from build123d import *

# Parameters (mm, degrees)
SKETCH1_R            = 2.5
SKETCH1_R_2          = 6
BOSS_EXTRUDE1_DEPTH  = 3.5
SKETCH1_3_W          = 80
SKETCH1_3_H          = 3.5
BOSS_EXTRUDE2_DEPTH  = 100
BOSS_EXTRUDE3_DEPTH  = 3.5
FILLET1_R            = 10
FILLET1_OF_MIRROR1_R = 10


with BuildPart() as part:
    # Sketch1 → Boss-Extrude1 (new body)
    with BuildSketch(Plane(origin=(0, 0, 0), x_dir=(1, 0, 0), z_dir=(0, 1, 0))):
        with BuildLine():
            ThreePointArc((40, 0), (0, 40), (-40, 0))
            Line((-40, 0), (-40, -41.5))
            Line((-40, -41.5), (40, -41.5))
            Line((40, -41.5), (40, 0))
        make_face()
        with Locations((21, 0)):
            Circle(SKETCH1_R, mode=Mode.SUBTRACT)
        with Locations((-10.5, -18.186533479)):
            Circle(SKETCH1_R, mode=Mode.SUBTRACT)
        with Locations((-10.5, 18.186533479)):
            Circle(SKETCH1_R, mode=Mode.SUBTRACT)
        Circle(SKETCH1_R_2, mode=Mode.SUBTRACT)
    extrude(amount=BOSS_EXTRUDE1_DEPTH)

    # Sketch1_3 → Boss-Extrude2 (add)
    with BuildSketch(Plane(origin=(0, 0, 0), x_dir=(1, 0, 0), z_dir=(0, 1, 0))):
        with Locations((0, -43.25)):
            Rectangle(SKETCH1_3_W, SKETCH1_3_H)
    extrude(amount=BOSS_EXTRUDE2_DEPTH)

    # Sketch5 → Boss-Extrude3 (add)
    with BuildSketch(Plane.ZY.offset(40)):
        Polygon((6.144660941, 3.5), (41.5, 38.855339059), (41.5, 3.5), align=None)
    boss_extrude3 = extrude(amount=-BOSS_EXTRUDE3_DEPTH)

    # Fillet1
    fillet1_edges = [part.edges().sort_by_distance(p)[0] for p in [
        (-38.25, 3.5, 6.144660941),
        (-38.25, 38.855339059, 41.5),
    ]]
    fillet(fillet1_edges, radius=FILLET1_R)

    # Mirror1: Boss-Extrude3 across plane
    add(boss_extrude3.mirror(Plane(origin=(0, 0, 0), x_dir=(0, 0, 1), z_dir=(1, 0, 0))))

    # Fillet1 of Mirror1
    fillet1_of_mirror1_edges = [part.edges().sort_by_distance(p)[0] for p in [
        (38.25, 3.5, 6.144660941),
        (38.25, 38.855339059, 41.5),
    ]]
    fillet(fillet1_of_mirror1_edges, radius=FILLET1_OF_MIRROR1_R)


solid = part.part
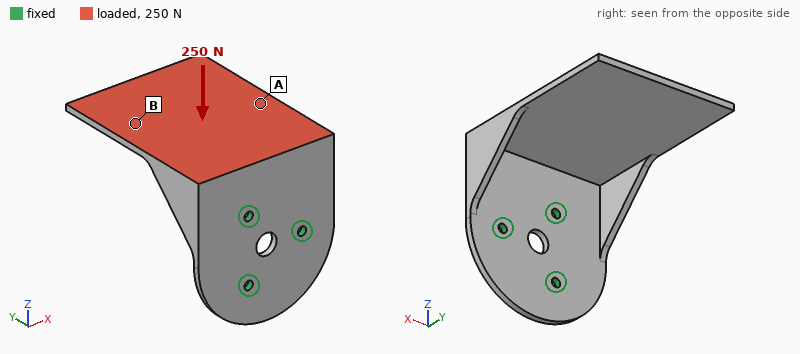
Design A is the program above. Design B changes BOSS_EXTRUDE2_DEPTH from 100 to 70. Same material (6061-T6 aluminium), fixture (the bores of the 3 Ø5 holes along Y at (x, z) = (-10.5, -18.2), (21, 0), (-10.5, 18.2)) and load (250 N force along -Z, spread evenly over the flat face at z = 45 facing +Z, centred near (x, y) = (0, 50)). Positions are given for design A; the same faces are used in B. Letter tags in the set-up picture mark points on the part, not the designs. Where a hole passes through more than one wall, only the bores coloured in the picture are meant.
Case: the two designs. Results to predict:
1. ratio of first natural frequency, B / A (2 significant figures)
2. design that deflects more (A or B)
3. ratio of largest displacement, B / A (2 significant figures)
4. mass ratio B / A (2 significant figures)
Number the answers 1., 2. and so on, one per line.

1. 1.7
2. A
3. 0.39
4. 0.84
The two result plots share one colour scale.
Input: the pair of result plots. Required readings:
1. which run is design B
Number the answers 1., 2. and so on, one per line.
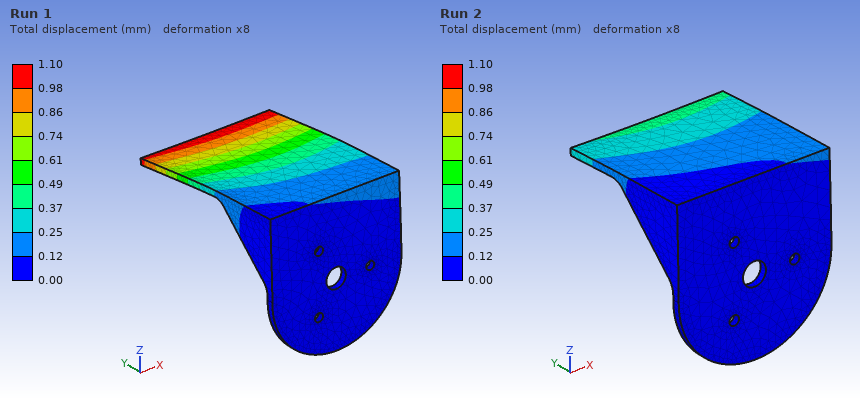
1. Run 2
